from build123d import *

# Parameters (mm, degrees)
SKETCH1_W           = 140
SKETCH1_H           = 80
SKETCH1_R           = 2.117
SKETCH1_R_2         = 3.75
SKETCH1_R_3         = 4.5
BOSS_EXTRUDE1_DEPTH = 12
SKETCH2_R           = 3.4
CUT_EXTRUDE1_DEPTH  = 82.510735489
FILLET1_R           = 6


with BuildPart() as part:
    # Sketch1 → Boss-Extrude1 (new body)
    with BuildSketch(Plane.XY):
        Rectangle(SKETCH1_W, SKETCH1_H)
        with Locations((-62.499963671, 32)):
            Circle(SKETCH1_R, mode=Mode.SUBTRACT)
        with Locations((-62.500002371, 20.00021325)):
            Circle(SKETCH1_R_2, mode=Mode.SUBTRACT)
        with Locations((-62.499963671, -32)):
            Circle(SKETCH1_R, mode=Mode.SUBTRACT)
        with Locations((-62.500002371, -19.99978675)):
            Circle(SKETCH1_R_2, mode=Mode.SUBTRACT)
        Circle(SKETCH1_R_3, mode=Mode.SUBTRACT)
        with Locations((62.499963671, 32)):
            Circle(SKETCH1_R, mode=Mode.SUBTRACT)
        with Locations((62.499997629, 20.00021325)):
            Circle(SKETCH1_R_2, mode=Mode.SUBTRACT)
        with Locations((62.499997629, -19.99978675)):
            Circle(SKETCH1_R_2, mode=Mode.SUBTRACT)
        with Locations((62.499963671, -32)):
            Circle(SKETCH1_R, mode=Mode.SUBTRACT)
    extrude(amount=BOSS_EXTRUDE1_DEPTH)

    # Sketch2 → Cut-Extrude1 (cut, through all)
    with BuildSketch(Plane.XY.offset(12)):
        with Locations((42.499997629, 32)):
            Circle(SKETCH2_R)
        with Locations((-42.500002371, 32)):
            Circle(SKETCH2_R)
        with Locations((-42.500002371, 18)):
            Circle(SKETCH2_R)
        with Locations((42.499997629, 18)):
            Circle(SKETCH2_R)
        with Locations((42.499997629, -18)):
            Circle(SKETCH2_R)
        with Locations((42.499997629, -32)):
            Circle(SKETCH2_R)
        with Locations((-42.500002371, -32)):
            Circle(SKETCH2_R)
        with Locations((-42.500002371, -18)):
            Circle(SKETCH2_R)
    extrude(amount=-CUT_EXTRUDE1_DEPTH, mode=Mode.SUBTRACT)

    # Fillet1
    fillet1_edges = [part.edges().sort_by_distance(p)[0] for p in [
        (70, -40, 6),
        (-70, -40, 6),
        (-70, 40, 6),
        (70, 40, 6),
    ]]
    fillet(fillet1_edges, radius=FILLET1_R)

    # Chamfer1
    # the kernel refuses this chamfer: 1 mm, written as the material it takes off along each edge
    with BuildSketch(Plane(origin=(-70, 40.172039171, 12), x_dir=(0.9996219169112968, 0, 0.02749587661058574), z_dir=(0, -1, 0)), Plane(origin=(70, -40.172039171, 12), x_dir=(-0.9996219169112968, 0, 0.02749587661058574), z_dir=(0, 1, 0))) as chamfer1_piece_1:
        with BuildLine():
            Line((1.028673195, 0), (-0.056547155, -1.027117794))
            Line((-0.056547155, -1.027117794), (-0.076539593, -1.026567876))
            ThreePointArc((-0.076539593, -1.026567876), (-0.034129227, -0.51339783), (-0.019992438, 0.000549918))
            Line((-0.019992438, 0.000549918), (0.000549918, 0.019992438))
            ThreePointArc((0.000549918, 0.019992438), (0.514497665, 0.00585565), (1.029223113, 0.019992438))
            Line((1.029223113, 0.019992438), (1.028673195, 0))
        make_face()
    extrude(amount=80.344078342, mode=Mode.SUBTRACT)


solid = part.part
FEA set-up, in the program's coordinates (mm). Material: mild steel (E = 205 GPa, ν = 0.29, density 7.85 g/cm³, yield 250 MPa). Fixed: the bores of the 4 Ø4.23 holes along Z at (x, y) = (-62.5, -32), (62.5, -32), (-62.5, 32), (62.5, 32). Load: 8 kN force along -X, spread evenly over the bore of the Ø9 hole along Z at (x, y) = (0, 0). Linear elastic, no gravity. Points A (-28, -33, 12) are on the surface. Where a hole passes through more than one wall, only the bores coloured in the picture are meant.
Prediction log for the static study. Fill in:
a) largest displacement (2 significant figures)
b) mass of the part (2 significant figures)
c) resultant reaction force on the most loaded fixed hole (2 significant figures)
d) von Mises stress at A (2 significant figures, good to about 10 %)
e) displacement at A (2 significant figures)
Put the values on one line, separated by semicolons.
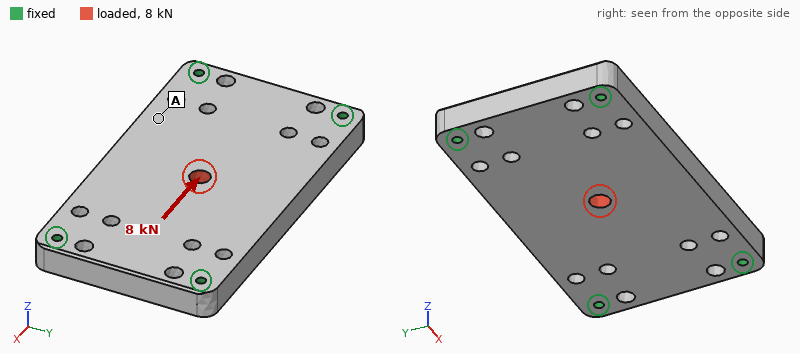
3.5 µm; 1000 g; 2.1 kN; 3.9 MPa; 1.4 µm
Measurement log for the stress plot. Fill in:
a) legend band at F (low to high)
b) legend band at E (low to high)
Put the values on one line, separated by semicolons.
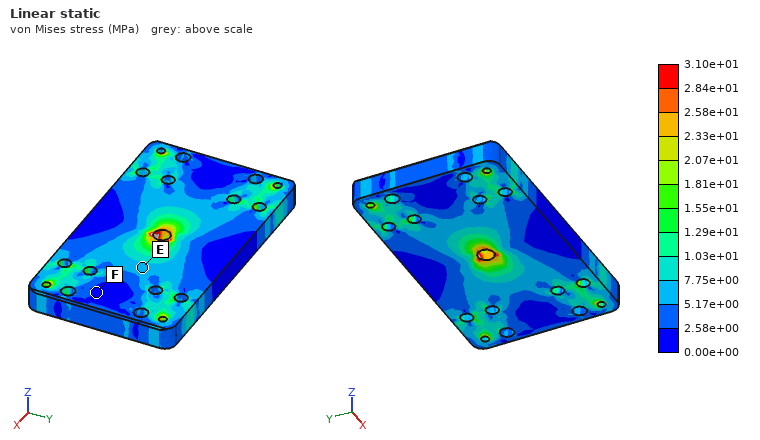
0.00e+00 to 2.58e+00 MPa; 5.17e+00 to 7.75e+00 MPa
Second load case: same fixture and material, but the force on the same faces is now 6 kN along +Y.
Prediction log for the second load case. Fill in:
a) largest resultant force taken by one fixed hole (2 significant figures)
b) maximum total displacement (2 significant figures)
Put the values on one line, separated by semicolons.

2.0 kN; 4.8 µm
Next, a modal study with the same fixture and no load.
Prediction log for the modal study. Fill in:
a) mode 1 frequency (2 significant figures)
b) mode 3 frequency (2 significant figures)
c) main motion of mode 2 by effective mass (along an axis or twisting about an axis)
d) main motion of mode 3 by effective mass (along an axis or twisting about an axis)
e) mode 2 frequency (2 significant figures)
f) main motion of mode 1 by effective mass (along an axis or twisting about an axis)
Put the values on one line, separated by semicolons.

3000 Hz; 7800 Hz; twisting about X; twisting about Y; 4900 Hz; along Z
